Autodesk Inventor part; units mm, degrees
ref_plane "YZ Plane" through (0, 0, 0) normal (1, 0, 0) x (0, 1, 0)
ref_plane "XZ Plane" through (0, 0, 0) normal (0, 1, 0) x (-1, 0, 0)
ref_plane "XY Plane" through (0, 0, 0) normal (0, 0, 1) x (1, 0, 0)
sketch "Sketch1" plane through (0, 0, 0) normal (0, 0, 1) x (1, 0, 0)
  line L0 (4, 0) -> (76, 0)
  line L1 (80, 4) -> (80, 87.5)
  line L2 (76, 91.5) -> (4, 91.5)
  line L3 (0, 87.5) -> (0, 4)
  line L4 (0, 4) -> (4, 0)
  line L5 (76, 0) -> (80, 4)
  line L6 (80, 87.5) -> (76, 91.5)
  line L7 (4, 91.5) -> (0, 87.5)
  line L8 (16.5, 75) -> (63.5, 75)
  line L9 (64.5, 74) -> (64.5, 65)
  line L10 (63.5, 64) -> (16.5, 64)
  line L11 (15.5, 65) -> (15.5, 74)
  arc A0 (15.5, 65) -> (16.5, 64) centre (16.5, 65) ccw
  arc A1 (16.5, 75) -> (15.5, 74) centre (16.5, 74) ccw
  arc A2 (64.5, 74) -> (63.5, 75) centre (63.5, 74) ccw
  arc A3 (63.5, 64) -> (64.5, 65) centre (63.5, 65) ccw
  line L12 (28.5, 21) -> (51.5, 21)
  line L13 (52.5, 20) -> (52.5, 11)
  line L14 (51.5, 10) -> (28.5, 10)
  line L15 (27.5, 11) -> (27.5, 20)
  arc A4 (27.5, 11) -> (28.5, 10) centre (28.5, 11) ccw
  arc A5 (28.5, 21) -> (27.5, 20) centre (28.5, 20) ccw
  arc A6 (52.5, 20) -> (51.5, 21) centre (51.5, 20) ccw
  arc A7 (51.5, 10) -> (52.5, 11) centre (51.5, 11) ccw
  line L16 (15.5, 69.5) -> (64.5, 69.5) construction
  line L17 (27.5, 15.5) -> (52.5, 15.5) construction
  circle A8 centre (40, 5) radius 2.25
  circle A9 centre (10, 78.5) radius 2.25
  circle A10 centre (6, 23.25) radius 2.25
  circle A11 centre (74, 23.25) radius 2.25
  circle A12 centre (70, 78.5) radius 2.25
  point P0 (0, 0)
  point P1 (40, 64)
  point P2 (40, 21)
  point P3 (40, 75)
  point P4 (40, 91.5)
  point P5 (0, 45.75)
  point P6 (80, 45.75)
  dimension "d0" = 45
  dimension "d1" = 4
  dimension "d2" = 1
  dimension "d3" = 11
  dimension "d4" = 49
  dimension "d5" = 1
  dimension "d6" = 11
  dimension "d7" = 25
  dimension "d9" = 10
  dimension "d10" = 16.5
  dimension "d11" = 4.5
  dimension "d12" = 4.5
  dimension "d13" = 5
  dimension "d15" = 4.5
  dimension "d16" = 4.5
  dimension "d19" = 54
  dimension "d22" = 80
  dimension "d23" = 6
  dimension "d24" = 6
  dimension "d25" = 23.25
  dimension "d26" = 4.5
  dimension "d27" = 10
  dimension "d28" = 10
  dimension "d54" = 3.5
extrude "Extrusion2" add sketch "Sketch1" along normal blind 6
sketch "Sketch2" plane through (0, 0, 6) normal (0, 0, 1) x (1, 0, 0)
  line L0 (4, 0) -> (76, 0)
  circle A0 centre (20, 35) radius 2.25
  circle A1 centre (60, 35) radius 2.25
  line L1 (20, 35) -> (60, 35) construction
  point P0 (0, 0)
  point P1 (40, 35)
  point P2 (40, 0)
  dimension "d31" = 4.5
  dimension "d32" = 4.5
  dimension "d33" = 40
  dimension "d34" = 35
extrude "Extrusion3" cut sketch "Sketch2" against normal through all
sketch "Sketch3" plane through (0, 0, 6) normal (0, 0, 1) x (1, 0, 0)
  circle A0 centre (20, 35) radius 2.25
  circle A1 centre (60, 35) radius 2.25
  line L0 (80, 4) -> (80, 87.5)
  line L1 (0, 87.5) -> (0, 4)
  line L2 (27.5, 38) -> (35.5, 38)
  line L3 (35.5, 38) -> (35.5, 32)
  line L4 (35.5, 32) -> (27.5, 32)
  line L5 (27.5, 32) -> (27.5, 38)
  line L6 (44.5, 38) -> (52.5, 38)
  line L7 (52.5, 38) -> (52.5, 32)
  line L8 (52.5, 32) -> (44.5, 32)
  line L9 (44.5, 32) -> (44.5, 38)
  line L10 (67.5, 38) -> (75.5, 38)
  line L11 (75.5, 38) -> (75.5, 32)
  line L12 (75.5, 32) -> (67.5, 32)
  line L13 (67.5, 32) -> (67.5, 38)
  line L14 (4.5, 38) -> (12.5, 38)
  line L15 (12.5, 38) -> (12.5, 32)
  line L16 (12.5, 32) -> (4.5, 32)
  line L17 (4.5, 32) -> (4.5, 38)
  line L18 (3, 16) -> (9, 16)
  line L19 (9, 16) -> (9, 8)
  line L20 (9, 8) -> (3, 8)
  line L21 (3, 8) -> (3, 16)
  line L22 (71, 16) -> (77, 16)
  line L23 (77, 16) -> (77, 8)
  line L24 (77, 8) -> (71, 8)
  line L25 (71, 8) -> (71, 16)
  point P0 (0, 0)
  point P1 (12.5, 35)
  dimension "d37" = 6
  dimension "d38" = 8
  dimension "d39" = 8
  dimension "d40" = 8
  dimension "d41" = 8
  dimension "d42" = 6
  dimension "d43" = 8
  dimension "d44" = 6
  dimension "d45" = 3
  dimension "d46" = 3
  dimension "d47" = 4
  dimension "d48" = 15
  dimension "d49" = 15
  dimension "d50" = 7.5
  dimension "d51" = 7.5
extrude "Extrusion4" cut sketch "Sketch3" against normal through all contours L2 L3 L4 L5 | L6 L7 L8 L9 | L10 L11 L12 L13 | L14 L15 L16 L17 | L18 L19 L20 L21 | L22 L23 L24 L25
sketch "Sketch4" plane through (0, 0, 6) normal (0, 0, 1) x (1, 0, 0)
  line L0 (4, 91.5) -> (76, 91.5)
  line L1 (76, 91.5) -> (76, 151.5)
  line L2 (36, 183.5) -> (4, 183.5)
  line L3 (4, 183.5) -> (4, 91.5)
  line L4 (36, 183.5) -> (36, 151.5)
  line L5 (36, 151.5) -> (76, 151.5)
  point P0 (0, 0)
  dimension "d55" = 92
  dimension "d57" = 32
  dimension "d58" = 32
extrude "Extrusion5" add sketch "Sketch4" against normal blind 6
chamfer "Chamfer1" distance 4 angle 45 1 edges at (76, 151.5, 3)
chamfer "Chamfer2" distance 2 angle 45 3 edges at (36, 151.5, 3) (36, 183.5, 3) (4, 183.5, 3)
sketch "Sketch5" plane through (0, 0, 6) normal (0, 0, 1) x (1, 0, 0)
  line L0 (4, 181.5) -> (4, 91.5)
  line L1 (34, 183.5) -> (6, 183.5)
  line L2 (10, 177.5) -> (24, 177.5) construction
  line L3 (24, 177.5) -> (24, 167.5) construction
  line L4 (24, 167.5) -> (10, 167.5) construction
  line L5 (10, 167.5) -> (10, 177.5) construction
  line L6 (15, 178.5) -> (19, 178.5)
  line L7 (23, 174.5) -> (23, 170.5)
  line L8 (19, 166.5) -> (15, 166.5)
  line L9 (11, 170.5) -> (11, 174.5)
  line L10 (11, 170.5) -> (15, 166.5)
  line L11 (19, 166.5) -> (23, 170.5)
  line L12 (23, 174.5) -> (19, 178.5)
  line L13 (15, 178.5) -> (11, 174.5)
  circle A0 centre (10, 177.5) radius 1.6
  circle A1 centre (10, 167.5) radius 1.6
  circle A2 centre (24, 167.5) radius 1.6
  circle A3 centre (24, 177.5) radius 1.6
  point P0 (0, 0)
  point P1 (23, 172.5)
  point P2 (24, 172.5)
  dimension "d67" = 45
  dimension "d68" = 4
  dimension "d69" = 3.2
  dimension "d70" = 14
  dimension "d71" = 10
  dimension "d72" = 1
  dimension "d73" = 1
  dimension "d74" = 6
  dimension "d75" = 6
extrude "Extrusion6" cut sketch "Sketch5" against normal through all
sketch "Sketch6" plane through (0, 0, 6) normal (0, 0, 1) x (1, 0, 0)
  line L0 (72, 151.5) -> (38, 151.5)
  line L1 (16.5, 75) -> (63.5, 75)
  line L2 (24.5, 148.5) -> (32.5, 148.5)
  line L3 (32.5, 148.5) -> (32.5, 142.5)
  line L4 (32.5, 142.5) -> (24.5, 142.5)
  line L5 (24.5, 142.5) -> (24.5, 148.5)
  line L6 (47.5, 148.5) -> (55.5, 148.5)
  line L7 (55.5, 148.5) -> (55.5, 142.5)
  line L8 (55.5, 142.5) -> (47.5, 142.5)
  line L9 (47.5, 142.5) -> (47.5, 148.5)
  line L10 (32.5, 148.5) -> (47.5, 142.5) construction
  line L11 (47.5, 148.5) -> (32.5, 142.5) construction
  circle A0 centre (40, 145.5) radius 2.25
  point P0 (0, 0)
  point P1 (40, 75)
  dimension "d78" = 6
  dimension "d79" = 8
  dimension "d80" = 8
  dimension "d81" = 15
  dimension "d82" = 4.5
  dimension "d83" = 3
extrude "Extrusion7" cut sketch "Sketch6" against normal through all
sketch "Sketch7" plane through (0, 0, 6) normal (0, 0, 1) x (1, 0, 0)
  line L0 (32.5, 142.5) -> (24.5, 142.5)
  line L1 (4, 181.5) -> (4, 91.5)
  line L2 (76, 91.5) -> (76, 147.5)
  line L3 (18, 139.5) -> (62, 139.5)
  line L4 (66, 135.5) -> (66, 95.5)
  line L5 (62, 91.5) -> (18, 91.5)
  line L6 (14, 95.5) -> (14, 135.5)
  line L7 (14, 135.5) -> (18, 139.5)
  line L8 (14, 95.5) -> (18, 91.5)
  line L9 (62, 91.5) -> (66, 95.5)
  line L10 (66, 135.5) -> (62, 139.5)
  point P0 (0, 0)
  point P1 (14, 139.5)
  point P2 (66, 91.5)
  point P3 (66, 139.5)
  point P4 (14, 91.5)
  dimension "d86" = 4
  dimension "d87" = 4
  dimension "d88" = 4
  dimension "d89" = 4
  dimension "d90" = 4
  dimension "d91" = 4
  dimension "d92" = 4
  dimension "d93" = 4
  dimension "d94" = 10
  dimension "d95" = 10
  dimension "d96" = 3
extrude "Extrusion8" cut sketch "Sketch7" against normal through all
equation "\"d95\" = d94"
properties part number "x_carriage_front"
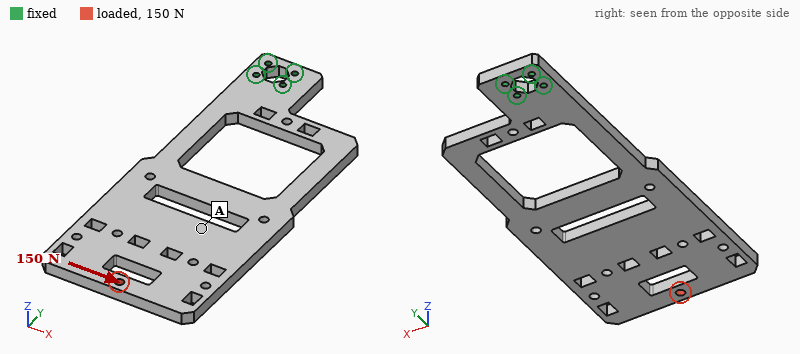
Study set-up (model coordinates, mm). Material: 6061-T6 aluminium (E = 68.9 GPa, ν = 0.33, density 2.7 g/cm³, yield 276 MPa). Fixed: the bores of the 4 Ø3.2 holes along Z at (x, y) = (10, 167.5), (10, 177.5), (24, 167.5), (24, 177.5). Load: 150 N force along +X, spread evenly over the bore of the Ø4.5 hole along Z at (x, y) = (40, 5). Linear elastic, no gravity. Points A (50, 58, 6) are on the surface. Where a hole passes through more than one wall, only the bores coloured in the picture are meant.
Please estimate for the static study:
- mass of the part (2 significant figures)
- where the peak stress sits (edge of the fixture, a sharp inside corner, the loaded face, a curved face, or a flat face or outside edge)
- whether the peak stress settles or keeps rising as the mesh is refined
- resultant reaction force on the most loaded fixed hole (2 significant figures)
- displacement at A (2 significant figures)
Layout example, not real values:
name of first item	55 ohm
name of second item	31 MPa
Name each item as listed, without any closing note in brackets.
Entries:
mass of the part	140 g
where the peak stress sits	a sharp inside corner
whether the peak stress settles or keeps rising as the mesh is refined	keeps rising
resultant reaction force on the most loaded fixed hole	1.1 kN
displacement at A	0.26 mm
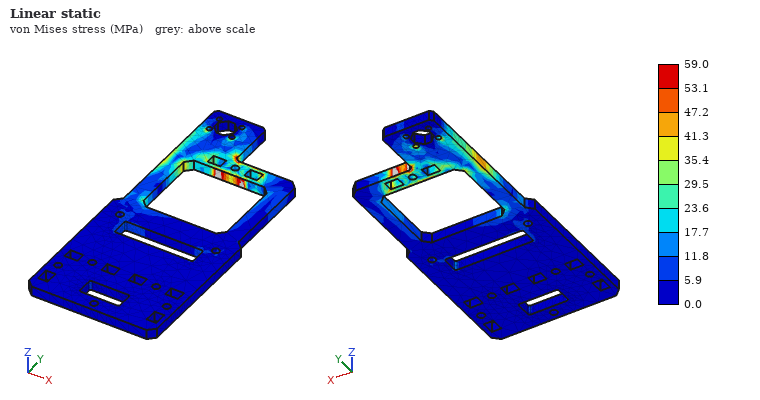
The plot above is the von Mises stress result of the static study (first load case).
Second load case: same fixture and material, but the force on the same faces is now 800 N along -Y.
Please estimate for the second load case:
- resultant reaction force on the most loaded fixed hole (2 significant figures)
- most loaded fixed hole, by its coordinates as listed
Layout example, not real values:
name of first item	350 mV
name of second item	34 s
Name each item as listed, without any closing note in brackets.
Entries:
resultant reaction force on the most loaded fixed hole	1.1 kN
most loaded fixed hole, by its coordinates as listed	(24, 167.5)
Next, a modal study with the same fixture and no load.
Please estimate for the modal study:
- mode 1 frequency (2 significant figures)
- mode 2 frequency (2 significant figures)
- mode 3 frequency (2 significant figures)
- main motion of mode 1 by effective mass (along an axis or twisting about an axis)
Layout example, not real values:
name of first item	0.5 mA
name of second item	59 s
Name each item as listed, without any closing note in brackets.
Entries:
mode 1 frequency	96 Hz
mode 2 frequency	400 Hz
mode 3 frequency	410 Hz
main motion of mode 1 by effective mass	along Z
